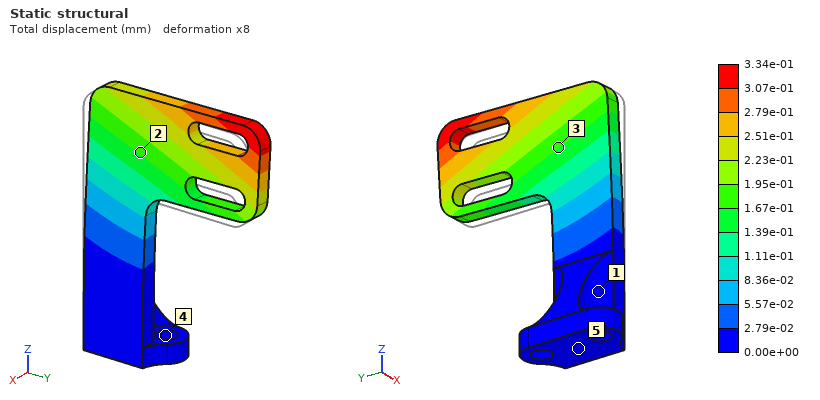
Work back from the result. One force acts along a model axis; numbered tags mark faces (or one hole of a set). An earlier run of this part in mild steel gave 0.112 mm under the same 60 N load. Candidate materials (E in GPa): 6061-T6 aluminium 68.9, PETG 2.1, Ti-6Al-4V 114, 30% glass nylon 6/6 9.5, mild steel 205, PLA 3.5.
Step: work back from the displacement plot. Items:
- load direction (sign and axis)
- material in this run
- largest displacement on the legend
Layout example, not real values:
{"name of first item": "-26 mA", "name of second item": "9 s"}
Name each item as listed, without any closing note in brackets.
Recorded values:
{"load direction": "-X", "material in this run": "6061-T6 aluminium", "largest displacement on the legend": "3.34e-01 mm"}
